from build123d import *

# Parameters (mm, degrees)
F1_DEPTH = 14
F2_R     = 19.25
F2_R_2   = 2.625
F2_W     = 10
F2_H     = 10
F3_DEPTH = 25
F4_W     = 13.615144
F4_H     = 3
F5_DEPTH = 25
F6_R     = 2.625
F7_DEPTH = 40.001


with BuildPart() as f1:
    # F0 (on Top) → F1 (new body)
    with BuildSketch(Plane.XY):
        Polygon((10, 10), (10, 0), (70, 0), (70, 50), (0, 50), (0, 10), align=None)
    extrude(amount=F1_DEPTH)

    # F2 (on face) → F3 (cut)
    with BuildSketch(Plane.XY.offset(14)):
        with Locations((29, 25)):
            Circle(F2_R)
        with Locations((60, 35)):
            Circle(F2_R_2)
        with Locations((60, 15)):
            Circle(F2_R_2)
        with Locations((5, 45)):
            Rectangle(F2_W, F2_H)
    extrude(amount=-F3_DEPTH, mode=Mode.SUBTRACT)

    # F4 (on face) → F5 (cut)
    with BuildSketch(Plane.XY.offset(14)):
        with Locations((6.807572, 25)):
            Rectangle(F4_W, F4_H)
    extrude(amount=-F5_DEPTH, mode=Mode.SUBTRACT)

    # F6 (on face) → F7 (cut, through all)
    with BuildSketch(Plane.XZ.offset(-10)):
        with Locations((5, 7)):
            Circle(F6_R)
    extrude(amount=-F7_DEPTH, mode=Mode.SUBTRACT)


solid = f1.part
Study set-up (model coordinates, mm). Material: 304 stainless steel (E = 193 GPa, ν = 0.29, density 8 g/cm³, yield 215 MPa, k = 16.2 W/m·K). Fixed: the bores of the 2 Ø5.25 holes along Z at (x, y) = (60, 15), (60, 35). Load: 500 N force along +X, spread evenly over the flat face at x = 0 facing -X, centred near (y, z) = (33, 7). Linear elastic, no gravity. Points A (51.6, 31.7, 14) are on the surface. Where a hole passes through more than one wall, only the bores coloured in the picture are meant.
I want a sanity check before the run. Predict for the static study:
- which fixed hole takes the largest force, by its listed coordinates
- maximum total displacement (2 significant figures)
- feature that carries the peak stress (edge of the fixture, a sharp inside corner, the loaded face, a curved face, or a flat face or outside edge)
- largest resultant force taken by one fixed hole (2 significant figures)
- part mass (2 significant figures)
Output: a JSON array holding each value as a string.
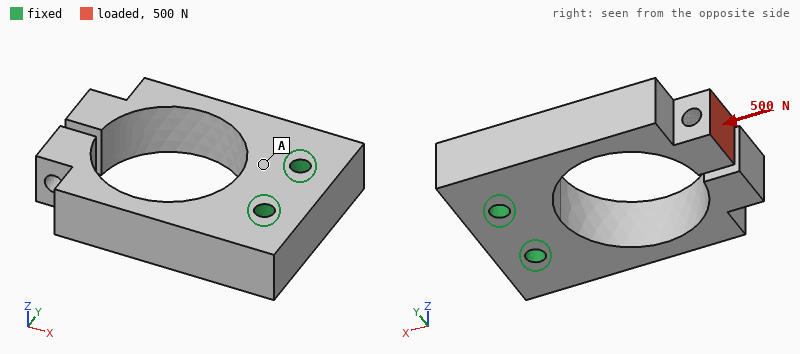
["(60, 35)", "0.11 mm", "a curved face", "450 N", "230 g"]
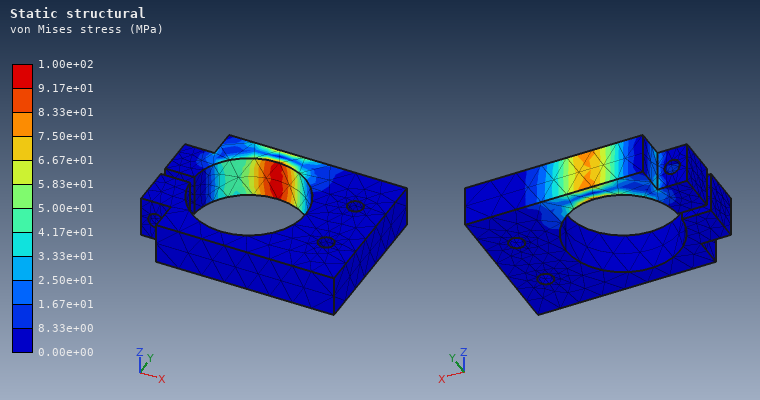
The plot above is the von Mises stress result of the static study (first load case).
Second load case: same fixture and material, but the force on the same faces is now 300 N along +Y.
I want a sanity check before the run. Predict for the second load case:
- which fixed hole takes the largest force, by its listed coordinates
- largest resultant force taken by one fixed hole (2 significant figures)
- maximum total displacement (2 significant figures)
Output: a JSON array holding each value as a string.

["(60, 15)", "720 N", "0.16 mm"]
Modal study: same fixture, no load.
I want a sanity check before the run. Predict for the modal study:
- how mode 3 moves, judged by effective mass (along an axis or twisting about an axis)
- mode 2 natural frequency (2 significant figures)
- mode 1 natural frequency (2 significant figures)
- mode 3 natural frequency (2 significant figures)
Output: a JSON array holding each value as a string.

["along Z", "1900 Hz", "1900 Hz", "2600 Hz"]
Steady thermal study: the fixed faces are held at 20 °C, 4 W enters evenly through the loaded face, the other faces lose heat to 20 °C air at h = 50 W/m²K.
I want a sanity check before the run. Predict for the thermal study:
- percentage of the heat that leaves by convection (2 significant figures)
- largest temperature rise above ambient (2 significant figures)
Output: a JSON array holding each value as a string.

["82 %", "53 K"]
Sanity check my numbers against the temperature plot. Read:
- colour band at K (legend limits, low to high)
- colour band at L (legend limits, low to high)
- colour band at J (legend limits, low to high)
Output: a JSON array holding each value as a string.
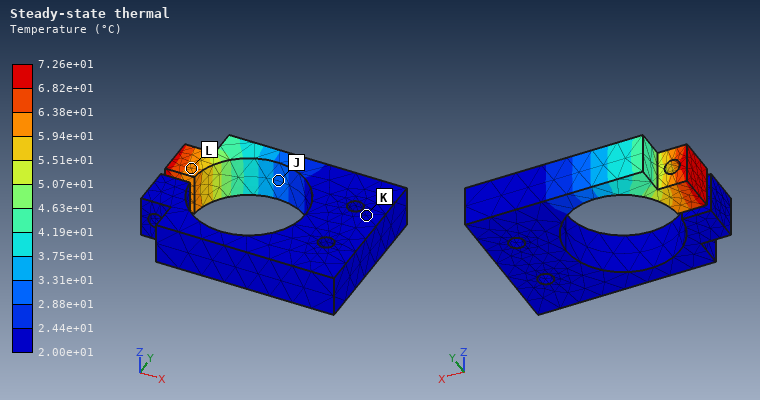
["2.00e+01 to 2.44e+01 °C", "5.94e+01 to 6.38e+01 °C", "2.88e+01 to 3.31e+01 °C"]
